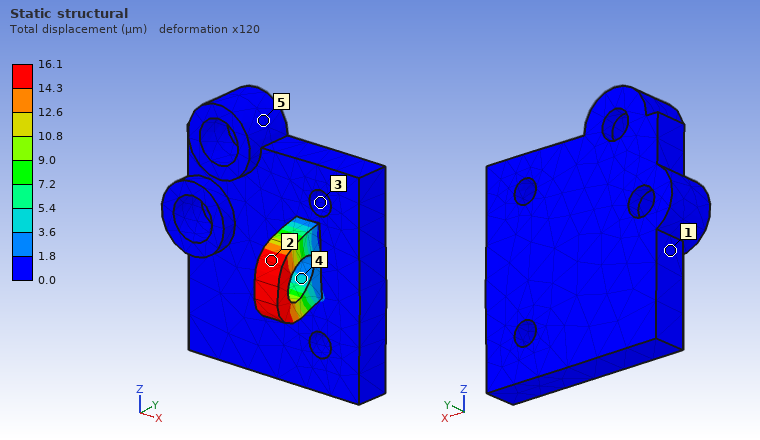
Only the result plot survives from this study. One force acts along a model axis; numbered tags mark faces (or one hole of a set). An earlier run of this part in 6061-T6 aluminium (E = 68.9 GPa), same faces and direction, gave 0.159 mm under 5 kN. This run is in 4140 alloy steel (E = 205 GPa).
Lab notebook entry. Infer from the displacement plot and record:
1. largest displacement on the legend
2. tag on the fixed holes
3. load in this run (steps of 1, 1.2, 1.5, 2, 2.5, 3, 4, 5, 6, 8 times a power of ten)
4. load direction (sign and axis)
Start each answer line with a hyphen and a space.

- 16.1 µm
- 3
- 1.5 kN
- -Z
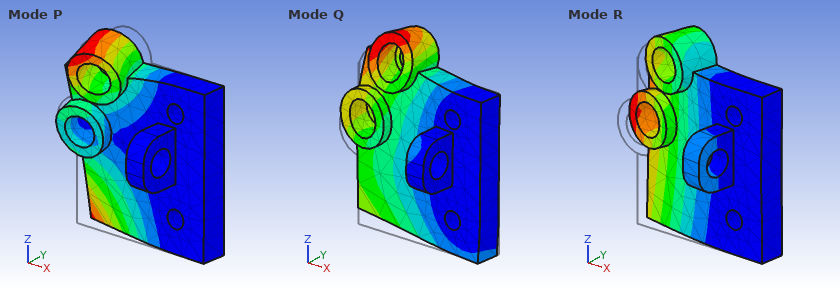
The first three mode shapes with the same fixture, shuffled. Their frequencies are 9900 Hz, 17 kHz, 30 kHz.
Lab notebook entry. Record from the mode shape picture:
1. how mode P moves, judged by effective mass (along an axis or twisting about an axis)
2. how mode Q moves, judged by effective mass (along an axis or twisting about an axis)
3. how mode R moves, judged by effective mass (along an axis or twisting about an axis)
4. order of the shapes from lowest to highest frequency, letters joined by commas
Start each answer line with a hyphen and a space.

- twisting about X
- along Z
- along Y
- R, P, Q
